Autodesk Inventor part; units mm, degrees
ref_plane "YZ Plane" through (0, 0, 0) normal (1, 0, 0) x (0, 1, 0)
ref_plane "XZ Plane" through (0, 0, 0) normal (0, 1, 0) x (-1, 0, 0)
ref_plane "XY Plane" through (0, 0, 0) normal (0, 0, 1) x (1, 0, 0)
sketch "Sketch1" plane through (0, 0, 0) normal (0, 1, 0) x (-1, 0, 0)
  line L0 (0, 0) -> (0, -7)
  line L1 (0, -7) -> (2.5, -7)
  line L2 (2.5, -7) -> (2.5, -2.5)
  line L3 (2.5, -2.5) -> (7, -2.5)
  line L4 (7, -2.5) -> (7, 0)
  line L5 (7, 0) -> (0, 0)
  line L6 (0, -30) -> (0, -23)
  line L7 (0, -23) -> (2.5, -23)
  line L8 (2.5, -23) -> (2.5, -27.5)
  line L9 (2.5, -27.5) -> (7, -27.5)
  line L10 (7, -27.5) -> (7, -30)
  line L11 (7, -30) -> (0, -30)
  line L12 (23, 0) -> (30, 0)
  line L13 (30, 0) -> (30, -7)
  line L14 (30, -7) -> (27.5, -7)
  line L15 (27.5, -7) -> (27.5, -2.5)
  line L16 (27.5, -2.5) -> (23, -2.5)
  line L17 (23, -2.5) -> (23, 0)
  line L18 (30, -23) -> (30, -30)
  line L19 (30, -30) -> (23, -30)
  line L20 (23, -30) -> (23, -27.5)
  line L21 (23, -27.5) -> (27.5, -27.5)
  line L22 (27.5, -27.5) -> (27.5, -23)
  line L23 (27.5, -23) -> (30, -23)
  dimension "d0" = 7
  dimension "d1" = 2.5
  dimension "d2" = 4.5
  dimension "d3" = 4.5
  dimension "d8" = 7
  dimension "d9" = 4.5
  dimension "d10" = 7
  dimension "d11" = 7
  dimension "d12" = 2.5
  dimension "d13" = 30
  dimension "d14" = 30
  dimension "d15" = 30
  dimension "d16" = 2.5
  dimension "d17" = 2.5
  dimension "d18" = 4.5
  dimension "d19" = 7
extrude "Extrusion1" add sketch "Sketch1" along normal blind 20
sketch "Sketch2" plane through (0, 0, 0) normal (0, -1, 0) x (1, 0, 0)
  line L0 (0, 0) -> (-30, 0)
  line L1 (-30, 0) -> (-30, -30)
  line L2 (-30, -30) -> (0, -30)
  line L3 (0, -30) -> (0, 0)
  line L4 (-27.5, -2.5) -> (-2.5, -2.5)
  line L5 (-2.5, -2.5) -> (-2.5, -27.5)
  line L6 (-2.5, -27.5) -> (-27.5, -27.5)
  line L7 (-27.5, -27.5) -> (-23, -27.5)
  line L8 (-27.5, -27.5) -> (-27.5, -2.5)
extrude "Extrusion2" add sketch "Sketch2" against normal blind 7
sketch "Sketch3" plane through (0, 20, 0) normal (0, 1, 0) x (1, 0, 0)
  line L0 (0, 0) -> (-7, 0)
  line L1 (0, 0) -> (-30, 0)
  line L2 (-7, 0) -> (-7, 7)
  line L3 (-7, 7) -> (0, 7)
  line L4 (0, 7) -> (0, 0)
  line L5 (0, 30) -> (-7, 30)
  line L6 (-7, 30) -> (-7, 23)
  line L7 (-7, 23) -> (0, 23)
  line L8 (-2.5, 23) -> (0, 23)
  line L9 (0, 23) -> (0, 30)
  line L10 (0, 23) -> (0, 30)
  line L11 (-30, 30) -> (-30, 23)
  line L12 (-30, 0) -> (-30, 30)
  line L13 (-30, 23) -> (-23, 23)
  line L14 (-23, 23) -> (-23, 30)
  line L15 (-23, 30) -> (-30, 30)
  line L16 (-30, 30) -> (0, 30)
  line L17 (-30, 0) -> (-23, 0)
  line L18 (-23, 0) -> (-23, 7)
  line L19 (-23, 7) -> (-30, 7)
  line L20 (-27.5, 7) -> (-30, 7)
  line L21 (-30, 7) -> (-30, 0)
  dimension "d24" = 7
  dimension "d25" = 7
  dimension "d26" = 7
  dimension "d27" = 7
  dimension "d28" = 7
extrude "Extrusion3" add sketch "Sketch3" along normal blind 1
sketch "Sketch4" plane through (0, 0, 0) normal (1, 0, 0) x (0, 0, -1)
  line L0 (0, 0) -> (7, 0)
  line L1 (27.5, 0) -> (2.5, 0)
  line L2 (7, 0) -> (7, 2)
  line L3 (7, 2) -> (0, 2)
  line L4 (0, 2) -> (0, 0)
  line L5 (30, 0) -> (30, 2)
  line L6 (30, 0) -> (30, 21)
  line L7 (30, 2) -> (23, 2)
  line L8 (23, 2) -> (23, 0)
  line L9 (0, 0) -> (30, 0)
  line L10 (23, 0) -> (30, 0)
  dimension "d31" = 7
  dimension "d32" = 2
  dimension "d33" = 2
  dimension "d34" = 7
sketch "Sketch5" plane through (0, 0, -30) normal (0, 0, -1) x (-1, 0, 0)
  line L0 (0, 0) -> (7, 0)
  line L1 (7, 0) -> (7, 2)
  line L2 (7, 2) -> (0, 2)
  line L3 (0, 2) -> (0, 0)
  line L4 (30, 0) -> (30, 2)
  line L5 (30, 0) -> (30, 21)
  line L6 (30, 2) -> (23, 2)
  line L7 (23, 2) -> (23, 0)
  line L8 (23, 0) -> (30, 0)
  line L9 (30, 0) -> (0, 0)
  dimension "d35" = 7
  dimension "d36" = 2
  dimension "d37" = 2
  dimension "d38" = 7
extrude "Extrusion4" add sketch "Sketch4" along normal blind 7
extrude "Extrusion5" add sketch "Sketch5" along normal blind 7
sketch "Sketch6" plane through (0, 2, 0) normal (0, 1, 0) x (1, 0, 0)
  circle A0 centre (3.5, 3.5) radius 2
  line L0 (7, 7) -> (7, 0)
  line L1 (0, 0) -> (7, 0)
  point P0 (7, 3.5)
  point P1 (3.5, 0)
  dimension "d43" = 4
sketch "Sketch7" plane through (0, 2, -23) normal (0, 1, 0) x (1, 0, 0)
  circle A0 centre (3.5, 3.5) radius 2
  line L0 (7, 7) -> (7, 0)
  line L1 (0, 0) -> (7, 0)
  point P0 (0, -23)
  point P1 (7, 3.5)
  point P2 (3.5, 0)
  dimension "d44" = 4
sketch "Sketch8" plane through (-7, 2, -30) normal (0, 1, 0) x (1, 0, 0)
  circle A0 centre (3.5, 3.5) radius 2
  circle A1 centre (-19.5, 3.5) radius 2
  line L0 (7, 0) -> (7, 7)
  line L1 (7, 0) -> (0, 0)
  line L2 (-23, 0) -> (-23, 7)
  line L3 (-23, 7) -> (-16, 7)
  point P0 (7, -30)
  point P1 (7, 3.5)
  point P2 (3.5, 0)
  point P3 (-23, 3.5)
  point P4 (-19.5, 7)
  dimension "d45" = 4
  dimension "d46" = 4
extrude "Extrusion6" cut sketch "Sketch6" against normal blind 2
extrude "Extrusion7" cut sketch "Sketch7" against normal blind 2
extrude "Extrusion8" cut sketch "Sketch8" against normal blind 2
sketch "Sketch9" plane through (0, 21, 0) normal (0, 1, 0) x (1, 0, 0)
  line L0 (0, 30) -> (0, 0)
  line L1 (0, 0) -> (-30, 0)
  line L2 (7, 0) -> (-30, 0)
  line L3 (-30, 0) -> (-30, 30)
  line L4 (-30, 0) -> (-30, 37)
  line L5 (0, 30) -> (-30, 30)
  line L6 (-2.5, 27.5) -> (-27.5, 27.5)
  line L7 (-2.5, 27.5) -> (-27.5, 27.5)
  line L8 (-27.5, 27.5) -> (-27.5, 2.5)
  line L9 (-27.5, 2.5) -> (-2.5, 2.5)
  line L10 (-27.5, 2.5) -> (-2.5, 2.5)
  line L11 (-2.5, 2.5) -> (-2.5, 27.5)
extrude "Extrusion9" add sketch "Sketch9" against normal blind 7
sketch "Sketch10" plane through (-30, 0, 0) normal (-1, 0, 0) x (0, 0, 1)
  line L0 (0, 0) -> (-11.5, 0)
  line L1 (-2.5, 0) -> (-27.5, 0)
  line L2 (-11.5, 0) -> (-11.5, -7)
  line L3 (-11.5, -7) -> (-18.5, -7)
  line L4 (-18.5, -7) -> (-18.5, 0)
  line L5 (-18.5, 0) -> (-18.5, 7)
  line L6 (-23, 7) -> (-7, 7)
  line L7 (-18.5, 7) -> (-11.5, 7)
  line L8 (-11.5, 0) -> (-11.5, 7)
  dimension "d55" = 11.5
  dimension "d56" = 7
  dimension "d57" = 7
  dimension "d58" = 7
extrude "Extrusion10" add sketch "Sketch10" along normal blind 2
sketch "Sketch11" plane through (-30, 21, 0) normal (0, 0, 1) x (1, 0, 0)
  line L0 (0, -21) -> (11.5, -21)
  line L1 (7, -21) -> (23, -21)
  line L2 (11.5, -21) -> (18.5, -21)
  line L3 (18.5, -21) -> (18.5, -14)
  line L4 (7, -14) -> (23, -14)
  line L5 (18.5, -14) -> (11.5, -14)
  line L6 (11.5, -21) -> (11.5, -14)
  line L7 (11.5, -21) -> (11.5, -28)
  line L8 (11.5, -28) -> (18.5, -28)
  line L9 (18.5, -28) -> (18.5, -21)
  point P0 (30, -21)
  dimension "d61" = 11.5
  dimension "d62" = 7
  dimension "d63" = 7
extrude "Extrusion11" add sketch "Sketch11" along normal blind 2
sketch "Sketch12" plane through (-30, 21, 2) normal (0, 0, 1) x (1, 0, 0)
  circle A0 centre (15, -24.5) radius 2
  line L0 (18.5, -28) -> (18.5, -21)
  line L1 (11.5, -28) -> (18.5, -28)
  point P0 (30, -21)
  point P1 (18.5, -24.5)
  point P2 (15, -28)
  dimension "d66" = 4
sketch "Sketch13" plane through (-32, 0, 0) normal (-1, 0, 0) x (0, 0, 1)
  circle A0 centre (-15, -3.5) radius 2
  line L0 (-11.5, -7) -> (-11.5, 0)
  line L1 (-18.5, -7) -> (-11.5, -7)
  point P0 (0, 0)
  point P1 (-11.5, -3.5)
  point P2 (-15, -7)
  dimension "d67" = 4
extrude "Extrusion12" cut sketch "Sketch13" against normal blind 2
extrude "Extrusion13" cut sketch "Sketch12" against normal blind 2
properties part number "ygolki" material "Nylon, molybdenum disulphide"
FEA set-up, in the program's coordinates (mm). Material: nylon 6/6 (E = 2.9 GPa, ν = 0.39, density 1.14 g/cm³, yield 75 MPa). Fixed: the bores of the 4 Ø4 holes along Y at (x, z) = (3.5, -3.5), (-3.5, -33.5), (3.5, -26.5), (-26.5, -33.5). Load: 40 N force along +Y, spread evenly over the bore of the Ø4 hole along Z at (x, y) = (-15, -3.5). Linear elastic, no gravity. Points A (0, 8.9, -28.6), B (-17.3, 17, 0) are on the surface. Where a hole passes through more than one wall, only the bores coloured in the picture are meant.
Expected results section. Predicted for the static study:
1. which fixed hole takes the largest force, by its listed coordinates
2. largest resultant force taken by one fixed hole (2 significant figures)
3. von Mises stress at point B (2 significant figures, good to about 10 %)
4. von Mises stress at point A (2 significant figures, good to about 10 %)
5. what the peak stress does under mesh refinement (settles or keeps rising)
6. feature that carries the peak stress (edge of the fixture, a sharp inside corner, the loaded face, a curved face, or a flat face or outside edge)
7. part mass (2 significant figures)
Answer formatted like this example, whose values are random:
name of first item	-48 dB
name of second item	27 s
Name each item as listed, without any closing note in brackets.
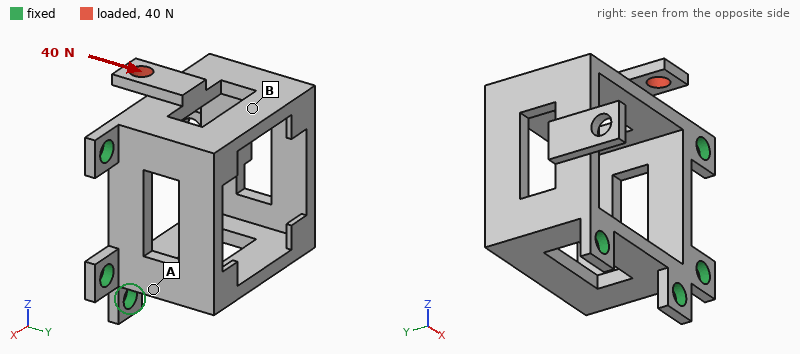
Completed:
which fixed hole takes the largest force, by its listed coordinates	(3.5, -3.5)
largest resultant force taken by one fixed hole	46 N
von Mises stress at point B	4.6 MPa
von Mises stress at point A	2.0 MPa
what the peak stress does under mesh refinement	keeps rising
feature that carries the peak stress	edge of the fixture
part mass	6.1 g
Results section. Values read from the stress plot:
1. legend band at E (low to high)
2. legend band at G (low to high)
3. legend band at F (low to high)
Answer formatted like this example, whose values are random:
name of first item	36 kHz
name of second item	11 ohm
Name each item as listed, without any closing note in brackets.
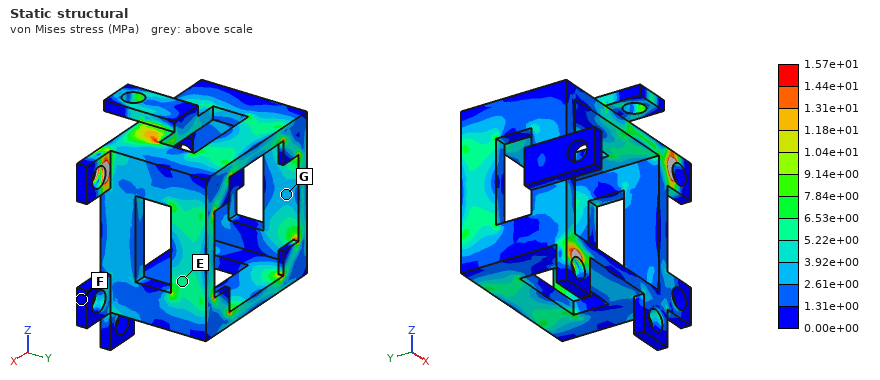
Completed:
legend band at E	5.22e+00 to 6.53e+00 MPa
legend band at G	2.61e+00 to 3.92e+00 MPa
legend band at F	0.00e+00 to 1.31e+00 MPa
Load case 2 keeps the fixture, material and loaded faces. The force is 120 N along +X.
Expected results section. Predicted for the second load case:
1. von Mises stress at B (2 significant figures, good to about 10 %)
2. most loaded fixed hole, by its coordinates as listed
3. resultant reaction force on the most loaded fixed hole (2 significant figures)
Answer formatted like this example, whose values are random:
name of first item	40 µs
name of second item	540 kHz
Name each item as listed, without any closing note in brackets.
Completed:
von Mises stress at B	6.4 MPa
most loaded fixed hole, by its coordinates as listed	(3.5, -3.5)
resultant reaction force on the most loaded fixed hole	130 N
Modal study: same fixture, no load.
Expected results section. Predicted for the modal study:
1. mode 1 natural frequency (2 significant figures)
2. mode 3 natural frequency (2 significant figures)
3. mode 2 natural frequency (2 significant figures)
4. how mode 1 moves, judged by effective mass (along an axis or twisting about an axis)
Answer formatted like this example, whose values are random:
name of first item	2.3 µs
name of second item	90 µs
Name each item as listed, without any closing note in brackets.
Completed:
mode 1 natural frequency	820 Hz
mode 3 natural frequency	3200 Hz
mode 2 natural frequency	2500 Hz
how mode 1 moves, judged by effective mass	along Y
